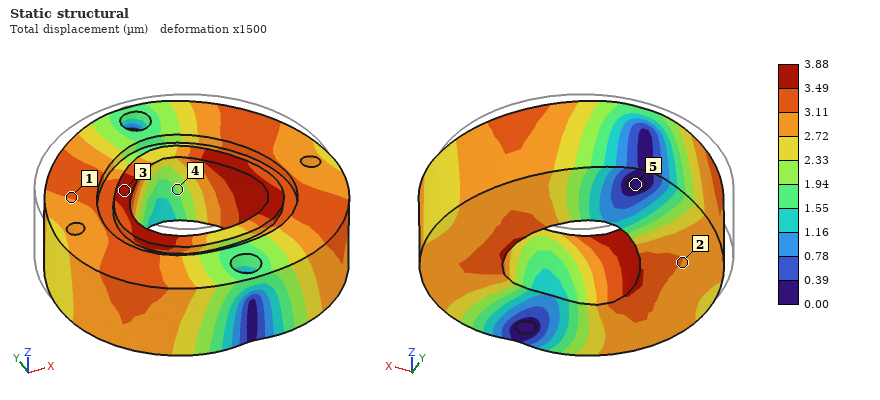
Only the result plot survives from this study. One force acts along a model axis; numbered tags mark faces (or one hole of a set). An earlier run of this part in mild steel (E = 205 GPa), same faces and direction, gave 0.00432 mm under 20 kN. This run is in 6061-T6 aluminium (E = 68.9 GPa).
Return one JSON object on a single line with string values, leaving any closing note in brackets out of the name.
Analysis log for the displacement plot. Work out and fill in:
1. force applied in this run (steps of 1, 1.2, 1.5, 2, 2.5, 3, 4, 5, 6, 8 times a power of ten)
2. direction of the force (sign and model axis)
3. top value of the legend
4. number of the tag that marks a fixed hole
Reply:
{"force applied in this run": "6 kN", "direction of the force": "-Y", "top value of the legend": "3.88 µm", "number of the tag that marks a fixed hole": "5"}
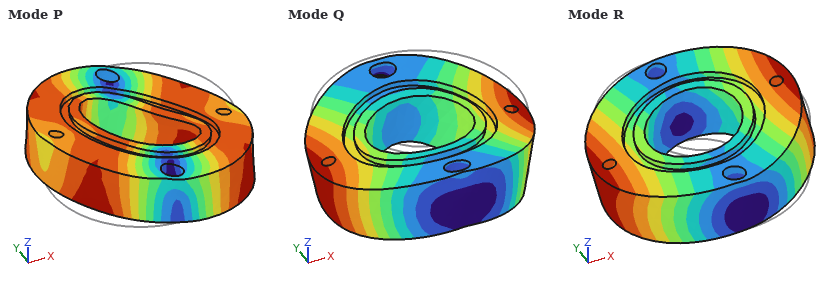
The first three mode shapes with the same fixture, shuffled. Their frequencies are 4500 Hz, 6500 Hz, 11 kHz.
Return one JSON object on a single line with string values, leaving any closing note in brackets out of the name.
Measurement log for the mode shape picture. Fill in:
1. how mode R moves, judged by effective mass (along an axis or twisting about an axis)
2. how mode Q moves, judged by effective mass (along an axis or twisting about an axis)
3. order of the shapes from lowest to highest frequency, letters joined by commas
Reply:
{"how mode R moves, judged by effective mass": "twisting about Y", "how mode Q moves, judged by effective mass": "along Z", "order of the shapes from lowest to highest frequency, letters joined by commas": "R, Q, P"}
